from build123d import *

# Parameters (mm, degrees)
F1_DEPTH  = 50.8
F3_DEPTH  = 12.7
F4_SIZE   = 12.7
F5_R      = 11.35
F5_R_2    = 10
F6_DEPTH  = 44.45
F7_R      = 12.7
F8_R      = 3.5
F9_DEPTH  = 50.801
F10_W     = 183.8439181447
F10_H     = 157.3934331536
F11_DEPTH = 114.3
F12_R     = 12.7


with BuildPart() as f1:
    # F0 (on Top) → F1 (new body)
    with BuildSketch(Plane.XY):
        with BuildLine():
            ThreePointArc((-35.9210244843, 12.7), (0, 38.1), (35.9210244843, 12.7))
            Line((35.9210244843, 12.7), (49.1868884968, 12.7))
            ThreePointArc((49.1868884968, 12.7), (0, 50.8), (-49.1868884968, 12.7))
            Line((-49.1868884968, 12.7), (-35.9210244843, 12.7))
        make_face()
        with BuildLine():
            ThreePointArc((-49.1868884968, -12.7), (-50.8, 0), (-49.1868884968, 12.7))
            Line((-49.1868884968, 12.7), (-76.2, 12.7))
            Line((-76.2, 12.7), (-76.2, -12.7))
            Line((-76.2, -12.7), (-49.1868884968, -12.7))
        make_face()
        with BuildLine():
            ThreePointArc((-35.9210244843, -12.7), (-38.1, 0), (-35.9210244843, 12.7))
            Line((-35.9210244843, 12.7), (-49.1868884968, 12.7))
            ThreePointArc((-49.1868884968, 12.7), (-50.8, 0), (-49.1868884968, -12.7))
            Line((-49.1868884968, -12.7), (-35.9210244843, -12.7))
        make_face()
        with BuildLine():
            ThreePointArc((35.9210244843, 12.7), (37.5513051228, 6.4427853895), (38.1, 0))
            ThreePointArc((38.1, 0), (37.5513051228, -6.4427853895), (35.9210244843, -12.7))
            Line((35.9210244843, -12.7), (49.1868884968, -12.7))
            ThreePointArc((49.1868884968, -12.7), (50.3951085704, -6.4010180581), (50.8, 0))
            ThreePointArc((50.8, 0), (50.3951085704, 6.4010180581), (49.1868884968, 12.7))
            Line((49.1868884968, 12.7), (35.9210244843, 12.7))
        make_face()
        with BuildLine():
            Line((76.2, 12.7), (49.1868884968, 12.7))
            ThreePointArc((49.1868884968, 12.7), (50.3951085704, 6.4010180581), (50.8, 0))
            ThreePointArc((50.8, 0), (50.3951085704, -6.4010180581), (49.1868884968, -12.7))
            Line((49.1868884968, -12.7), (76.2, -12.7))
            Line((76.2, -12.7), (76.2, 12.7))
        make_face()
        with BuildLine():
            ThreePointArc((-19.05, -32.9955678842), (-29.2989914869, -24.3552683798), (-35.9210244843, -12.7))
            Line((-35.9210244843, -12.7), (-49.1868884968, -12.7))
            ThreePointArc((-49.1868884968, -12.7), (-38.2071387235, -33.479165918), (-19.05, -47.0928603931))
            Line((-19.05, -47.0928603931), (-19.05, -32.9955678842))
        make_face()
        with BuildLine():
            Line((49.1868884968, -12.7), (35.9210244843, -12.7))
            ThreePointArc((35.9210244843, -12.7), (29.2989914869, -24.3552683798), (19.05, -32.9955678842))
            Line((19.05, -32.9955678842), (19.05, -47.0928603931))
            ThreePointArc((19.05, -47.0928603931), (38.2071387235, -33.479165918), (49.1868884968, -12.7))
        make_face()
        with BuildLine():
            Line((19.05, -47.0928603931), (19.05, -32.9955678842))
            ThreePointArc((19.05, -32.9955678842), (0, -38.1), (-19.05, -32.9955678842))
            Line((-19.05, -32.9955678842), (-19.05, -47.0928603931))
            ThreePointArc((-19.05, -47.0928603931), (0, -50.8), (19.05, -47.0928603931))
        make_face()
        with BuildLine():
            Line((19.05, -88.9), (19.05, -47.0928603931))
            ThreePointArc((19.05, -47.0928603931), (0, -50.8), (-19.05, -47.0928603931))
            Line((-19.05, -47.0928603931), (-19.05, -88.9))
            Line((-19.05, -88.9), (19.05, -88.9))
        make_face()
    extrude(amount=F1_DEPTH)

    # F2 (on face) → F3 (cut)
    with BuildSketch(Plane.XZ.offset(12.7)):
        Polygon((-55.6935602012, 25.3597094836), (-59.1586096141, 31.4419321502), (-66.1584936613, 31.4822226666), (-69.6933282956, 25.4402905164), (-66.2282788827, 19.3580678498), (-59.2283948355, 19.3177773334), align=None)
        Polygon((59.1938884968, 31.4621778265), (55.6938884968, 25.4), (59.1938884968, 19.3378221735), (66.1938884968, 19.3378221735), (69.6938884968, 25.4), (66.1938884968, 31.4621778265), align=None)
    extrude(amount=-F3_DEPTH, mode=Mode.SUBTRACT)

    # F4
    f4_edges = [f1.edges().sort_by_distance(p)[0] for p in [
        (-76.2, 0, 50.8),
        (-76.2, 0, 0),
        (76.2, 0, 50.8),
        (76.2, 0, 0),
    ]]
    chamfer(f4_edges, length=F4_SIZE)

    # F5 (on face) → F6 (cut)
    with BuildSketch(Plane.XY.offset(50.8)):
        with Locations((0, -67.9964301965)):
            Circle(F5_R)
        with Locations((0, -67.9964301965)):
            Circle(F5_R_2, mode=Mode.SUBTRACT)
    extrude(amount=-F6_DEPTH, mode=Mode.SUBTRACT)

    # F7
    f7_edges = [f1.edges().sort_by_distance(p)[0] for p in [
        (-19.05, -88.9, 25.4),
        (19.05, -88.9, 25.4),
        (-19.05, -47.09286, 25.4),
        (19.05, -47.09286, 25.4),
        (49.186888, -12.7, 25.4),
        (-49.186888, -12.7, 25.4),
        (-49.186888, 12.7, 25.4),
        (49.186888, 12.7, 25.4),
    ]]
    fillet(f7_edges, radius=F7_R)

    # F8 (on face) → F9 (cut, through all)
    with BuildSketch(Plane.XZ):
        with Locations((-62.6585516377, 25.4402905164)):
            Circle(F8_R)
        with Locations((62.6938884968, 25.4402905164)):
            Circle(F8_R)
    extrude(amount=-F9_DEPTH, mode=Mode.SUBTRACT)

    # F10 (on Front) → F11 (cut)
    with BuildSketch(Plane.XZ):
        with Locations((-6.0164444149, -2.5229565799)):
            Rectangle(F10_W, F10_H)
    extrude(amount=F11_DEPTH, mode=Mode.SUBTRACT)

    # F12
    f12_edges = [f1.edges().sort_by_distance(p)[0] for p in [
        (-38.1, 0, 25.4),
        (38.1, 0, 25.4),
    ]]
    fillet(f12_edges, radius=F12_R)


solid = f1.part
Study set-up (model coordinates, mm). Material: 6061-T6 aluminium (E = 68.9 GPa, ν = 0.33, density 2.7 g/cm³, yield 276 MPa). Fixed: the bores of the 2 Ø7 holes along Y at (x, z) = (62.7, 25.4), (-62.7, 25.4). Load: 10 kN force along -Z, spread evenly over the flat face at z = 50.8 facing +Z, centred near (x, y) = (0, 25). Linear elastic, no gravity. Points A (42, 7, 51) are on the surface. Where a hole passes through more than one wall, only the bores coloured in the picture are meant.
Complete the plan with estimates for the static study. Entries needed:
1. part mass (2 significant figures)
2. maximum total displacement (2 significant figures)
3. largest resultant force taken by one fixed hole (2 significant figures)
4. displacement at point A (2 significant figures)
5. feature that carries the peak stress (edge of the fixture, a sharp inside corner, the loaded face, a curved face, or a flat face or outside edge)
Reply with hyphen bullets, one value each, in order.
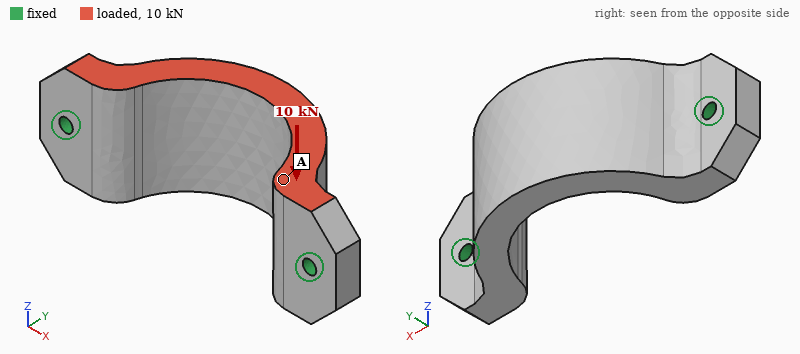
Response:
- 320 g
- 0.22 mm
- 5.0 kN
- 0.085 mm
- edge of the fixture
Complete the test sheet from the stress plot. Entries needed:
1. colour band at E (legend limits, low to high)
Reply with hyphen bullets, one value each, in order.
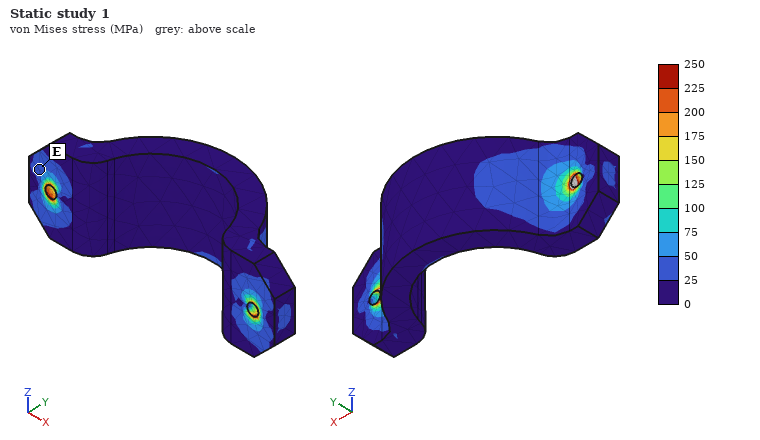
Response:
- 25 to 50 MPa
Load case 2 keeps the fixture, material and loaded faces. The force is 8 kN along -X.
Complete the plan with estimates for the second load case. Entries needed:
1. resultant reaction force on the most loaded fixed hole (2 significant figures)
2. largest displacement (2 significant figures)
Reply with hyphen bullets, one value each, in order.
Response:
- 4.3 kN
- 49 µm
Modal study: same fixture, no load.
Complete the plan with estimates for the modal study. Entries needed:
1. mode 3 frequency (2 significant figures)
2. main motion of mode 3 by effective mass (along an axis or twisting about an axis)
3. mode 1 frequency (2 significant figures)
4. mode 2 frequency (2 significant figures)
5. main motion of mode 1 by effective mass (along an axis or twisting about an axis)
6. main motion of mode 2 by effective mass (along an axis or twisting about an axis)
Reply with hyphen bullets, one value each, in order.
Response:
- 6700 Hz
- along Y
- 2400 Hz
- 5700 Hz
- along Z
- along X
